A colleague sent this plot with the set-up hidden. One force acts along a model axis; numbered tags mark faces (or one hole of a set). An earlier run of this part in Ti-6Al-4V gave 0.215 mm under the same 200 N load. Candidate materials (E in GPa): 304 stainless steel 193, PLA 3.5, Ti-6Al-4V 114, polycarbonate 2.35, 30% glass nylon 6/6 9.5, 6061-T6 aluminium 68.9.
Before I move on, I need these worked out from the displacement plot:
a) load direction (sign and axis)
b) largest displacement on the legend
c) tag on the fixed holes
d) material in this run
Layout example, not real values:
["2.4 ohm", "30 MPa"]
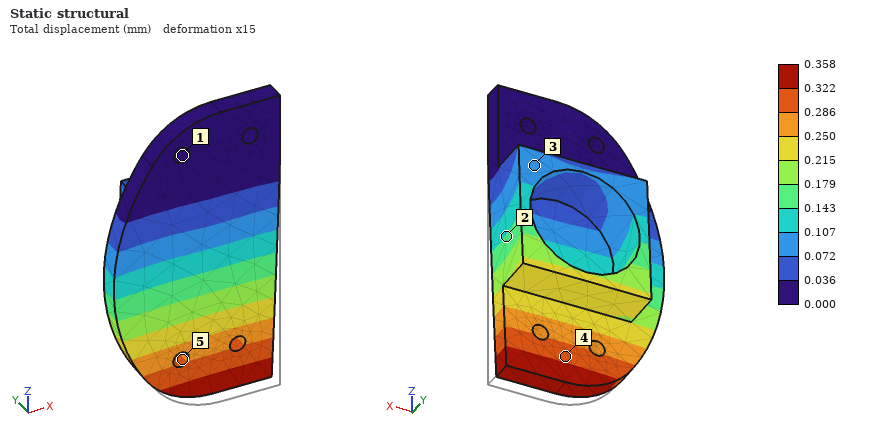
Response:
["+Y", "0.358 mm", "1", "6061-T6 aluminium"]
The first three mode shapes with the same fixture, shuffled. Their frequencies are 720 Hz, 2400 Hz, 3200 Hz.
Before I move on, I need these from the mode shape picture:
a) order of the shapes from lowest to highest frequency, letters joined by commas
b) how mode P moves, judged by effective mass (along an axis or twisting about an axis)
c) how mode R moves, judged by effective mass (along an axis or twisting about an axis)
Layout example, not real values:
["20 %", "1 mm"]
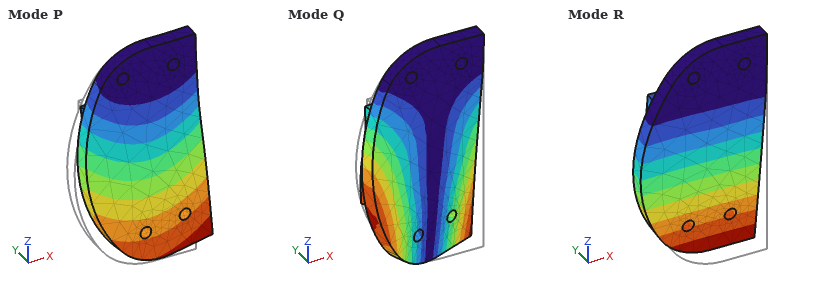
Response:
["R, Q, P", "along X", "along Y"]
